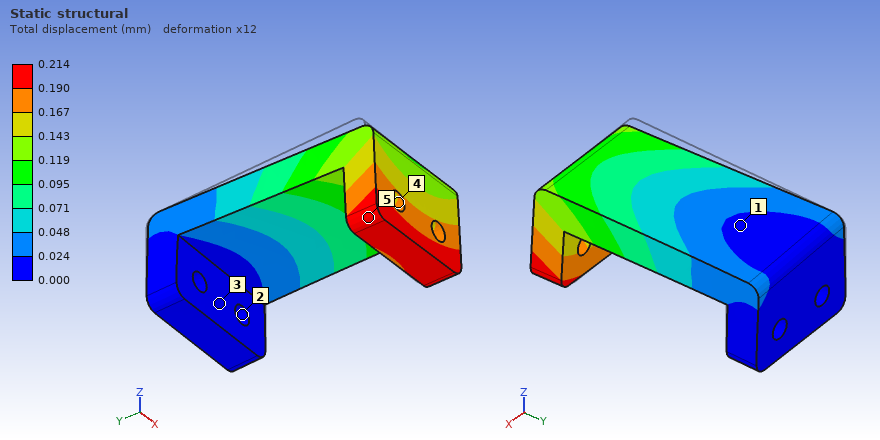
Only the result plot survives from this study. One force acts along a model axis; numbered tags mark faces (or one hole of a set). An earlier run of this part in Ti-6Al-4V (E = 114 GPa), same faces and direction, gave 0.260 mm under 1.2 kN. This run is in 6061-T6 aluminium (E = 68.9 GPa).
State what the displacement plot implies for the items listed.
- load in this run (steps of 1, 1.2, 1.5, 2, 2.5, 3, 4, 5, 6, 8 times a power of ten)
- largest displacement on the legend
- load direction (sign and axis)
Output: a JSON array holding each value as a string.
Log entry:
["600 N", "0.214 mm", "+X"]
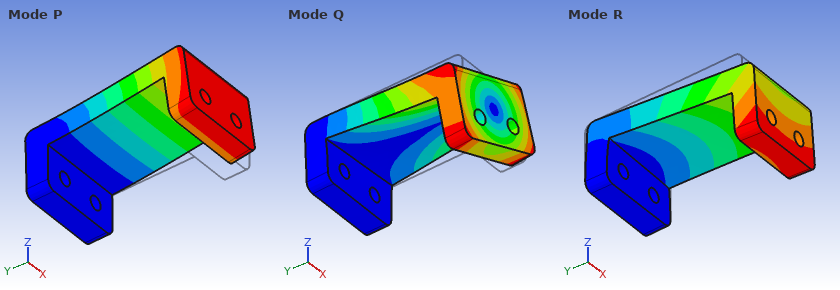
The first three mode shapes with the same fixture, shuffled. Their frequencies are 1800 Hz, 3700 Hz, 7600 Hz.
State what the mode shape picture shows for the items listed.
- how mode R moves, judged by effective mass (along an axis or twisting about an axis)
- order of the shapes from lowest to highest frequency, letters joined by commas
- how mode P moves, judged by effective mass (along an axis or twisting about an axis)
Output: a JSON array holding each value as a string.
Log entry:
["along X", "P, R, Q", "along Z"]
